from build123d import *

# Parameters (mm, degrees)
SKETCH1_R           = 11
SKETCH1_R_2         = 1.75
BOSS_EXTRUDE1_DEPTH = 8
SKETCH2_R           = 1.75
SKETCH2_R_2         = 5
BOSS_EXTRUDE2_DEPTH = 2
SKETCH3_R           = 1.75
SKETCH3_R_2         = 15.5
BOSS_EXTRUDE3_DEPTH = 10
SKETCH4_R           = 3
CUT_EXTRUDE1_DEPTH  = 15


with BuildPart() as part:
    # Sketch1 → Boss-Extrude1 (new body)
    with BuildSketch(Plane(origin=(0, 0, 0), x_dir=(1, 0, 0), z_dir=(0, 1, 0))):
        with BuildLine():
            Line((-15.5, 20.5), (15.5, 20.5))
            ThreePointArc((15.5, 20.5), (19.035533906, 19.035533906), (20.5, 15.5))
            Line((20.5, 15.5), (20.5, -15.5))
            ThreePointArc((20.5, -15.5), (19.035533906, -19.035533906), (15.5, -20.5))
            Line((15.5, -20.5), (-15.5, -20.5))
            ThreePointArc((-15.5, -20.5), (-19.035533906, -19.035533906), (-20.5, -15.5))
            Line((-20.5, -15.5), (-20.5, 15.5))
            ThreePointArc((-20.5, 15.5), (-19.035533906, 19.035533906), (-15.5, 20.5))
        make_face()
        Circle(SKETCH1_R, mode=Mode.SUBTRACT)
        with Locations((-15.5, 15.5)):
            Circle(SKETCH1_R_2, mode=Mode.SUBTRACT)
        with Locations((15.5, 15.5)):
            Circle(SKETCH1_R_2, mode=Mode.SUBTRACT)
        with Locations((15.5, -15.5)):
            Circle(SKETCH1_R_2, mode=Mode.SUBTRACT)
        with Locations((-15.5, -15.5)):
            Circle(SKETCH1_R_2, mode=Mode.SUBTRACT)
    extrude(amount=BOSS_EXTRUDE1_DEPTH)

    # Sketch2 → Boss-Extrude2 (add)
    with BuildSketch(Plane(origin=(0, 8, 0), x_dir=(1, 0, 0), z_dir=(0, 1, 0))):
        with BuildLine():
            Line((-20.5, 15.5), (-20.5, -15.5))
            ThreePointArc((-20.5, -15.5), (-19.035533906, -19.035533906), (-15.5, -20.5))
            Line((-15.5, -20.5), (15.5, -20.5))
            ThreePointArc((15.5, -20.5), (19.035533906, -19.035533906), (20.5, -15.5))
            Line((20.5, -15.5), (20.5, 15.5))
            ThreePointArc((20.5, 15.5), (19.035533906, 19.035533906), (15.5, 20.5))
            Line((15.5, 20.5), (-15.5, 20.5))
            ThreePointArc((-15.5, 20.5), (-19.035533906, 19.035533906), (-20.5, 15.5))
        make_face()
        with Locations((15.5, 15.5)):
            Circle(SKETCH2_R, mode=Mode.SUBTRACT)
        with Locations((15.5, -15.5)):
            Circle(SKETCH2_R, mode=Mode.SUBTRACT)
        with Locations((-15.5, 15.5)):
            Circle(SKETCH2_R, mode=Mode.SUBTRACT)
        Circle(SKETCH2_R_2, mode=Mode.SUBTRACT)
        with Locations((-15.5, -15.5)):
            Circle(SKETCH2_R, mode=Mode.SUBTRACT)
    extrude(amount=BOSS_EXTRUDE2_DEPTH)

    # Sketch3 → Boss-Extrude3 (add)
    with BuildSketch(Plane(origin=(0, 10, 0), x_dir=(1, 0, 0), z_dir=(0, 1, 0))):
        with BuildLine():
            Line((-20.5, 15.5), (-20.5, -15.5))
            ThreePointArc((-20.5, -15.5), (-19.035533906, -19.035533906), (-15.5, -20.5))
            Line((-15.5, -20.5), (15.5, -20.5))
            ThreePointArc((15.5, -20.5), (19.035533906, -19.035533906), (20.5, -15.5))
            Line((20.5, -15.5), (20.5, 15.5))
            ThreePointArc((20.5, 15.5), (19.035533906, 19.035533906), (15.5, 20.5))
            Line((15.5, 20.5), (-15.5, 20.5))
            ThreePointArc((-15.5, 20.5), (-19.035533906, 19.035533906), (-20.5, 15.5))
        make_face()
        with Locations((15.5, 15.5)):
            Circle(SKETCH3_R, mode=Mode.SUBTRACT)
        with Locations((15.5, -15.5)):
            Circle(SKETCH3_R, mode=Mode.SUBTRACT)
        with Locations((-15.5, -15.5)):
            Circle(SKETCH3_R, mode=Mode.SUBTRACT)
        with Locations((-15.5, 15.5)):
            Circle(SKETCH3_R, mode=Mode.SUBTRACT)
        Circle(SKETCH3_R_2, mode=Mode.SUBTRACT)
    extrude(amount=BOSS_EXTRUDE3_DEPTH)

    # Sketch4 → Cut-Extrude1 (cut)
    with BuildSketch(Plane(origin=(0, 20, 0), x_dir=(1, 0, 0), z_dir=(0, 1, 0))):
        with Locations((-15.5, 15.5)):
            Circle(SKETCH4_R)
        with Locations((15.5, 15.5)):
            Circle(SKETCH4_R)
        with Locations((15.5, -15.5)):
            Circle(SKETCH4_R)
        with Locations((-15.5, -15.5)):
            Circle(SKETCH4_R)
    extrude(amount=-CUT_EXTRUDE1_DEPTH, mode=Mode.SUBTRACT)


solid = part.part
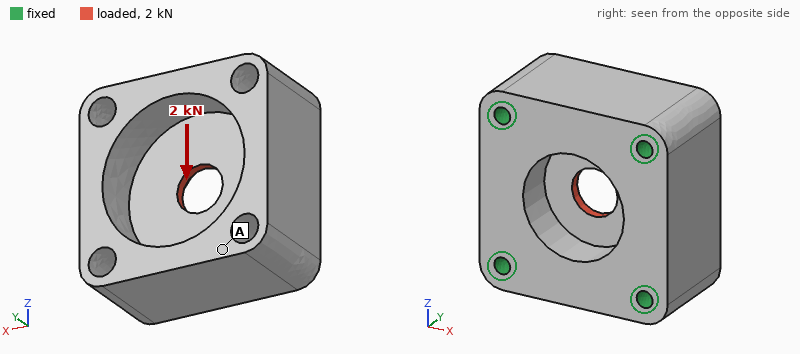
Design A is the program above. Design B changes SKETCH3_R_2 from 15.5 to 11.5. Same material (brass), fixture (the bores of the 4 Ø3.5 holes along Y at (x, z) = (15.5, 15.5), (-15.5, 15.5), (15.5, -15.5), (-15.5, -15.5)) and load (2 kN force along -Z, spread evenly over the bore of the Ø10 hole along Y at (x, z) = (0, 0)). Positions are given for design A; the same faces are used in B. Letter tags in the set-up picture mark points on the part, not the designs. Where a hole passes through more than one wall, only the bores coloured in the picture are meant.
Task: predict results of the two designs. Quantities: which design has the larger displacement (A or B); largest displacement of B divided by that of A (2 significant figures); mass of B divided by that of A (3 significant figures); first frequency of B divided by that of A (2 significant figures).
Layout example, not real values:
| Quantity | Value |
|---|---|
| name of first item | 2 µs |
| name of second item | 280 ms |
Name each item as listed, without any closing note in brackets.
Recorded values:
| Quantity | Value |
|---|---|
| which design has the larger displacement | A |
| largest displacement of B divided by that of A | 0.81 |
| mass of B divided by that of A | 1.17 |
| first frequency of B divided by that of A | 1.0 |
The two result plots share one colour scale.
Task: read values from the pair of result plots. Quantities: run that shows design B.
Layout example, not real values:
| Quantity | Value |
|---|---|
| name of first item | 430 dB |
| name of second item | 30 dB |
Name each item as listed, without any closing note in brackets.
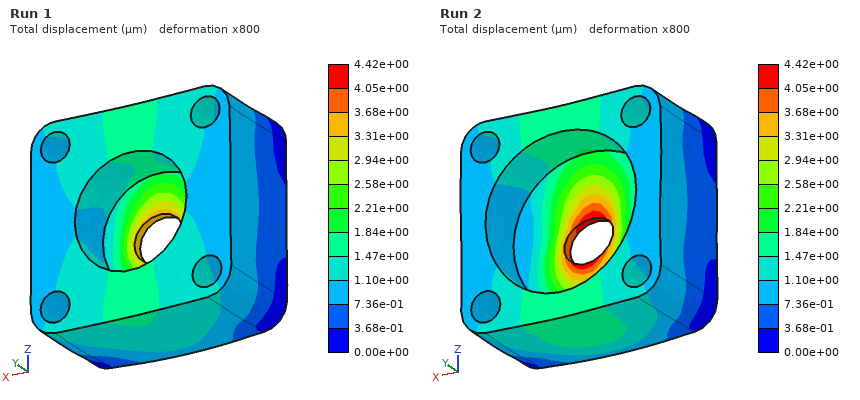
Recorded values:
| Quantity | Value |
|---|---|
| run that shows design B | Run 1 |
